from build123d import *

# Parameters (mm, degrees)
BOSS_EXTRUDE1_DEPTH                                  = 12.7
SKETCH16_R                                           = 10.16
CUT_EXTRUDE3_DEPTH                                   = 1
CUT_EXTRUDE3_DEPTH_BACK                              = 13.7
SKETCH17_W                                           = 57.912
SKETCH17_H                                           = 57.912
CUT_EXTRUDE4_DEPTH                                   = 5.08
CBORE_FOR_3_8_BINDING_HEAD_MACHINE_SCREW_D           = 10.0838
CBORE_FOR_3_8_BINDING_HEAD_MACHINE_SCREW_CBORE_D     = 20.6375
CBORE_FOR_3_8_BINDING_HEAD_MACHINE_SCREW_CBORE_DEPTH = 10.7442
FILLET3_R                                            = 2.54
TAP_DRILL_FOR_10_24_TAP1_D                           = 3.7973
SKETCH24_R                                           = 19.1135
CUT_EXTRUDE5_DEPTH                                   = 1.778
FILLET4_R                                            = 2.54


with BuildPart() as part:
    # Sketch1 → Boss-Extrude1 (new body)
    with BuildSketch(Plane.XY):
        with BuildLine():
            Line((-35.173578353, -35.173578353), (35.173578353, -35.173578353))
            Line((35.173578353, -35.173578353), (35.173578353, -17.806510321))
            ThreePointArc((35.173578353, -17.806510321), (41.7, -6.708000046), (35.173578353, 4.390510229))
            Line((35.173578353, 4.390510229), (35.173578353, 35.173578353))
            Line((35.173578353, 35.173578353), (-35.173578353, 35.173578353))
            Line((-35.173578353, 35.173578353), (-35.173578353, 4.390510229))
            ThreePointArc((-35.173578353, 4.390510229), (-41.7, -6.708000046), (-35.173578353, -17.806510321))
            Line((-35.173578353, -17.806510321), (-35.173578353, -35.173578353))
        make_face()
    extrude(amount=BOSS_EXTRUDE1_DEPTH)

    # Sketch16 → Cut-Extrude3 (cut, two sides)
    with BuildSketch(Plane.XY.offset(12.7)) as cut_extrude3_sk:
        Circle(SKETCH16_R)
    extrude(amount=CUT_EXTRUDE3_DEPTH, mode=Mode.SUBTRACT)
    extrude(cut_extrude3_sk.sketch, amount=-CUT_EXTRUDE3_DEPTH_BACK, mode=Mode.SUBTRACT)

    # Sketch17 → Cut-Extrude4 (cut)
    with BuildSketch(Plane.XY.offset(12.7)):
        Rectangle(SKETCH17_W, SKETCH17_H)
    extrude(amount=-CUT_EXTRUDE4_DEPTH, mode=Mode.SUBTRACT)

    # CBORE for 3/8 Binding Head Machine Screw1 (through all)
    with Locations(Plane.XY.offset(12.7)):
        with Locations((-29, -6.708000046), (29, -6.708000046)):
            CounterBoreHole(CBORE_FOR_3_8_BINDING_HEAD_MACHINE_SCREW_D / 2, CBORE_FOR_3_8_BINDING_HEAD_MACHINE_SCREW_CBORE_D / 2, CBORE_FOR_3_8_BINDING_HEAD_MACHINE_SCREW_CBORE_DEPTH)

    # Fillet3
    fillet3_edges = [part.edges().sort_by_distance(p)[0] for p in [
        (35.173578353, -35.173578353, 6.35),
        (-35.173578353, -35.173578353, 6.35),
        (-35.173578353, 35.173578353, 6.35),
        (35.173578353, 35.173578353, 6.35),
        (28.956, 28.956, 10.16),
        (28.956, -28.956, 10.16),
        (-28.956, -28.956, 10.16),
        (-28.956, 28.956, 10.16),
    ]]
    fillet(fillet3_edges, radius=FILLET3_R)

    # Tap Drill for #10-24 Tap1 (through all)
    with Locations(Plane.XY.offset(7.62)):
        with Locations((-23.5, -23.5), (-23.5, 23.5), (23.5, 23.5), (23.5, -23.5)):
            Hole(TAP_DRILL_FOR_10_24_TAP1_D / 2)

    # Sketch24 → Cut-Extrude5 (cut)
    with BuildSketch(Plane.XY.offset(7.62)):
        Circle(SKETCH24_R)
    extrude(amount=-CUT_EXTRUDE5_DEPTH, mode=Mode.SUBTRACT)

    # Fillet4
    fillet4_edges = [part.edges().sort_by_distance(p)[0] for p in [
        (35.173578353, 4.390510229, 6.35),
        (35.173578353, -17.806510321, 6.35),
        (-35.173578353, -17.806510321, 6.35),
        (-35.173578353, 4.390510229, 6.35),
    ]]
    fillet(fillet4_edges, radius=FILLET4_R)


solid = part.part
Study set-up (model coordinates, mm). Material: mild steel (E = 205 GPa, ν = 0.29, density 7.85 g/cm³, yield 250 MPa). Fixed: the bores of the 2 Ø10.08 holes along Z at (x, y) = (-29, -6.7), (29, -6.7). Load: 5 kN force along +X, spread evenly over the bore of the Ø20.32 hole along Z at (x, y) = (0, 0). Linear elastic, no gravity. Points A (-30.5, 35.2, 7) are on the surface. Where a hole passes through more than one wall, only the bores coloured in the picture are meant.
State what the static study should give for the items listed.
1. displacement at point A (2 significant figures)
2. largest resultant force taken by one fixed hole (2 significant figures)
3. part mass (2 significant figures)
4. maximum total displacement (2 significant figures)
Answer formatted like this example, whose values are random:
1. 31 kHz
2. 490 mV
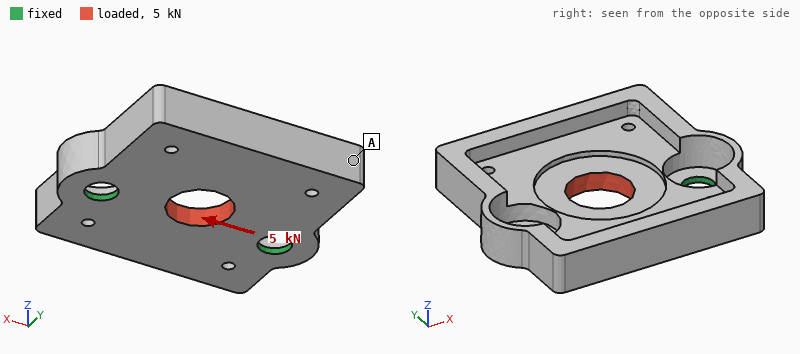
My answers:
1. 4.1 µm
2. 2.6 kN
3. 300 g
4. 4.8 µm
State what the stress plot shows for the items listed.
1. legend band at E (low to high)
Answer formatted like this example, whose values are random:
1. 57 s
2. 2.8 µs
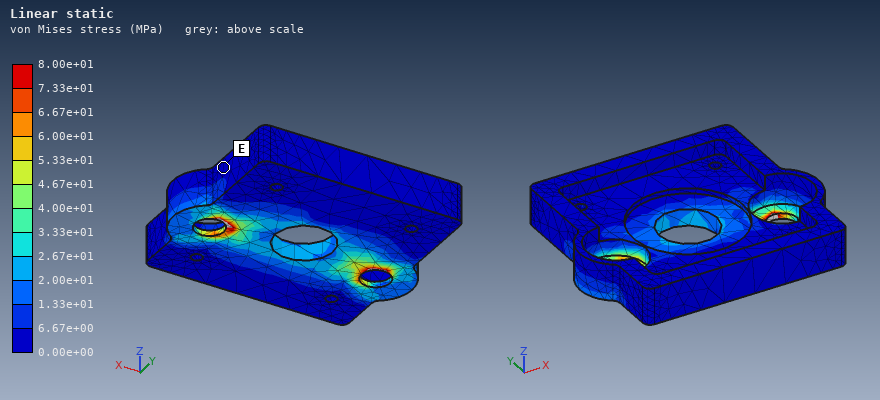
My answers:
1. 0.00e+00 to 6.67e+00 MPa
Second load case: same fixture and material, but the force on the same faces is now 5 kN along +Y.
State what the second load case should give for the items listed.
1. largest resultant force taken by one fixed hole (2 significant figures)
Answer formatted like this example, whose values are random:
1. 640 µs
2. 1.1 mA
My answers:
1. 2.5 kN
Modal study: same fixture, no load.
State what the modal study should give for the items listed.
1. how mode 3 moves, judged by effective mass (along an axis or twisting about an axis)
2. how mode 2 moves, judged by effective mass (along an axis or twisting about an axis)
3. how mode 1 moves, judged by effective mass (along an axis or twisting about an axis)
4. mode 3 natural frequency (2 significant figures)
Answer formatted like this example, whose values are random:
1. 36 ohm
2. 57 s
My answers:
1. twisting about Y
2. along Z
3. along Z
4. 3800 Hz
